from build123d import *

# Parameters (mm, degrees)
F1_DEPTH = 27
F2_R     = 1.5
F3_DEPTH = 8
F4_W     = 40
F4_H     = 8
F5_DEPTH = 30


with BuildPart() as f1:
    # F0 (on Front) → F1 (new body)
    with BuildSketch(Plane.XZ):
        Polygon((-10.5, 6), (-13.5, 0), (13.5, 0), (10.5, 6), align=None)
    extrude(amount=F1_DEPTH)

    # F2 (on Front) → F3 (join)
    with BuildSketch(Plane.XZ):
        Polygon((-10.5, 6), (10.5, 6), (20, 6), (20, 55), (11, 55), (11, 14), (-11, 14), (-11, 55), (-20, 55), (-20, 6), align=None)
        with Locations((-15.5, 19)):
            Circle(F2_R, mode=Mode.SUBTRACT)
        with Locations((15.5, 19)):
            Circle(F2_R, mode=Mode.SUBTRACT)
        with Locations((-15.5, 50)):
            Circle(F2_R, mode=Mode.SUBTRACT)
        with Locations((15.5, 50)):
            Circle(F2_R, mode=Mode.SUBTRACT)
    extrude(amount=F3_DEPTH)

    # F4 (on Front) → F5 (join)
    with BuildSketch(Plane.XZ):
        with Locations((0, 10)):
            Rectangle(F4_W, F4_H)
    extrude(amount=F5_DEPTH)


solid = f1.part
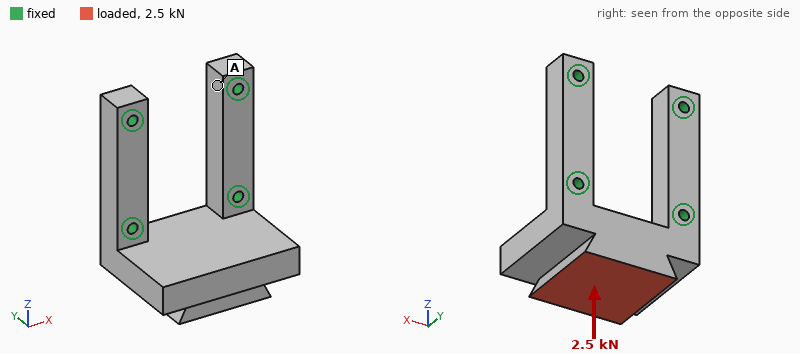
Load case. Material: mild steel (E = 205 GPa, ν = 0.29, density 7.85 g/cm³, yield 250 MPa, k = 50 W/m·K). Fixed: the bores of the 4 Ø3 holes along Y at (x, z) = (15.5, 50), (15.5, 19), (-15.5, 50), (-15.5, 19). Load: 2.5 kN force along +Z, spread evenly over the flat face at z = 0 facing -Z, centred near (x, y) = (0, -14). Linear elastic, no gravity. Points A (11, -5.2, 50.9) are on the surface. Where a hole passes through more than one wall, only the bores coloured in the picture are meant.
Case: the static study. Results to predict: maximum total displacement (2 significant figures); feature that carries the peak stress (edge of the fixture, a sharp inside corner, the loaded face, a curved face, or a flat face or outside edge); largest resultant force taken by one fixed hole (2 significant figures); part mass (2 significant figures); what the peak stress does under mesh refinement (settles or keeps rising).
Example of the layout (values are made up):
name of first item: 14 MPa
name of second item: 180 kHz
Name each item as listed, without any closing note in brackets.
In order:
maximum total displacement: 41 µm
feature that carries the peak stress: edge of the fixture
largest resultant force taken by one fixed hole: 1.3 kN
part mass: 150 g
what the peak stress does under mesh refinement: keeps rising
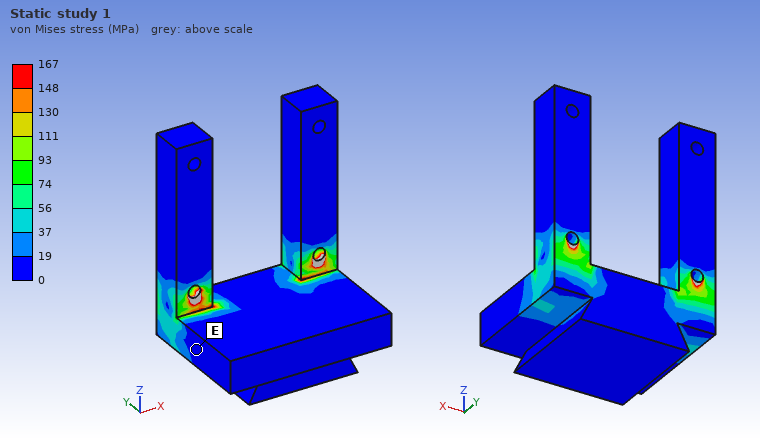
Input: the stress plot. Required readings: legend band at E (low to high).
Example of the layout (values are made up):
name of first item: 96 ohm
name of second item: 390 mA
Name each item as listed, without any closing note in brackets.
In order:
legend band at E: 0 to 19 MPa
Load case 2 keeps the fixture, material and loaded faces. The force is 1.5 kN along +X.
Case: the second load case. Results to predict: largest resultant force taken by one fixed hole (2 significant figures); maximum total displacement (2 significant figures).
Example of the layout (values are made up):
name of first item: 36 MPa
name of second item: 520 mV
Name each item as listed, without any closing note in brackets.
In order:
largest resultant force taken by one fixed hole: 1.2 kN
maximum total displacement: 4.2 µm
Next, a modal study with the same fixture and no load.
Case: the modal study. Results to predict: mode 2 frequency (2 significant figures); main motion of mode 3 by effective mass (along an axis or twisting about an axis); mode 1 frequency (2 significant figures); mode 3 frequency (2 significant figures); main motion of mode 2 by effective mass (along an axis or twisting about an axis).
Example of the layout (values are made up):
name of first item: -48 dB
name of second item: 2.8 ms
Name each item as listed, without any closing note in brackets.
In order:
mode 2 frequency: 10 kHz
main motion of mode 3 by effective mass: along Y
mode 1 frequency: 4000 Hz
mode 3 frequency: 15 kHz
main motion of mode 2 by effective mass: along X
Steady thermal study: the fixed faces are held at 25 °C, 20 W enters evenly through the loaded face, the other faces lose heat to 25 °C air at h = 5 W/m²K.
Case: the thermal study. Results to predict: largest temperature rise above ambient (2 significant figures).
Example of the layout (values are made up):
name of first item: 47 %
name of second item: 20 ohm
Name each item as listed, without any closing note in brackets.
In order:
largest temperature rise above ambient: 38 K
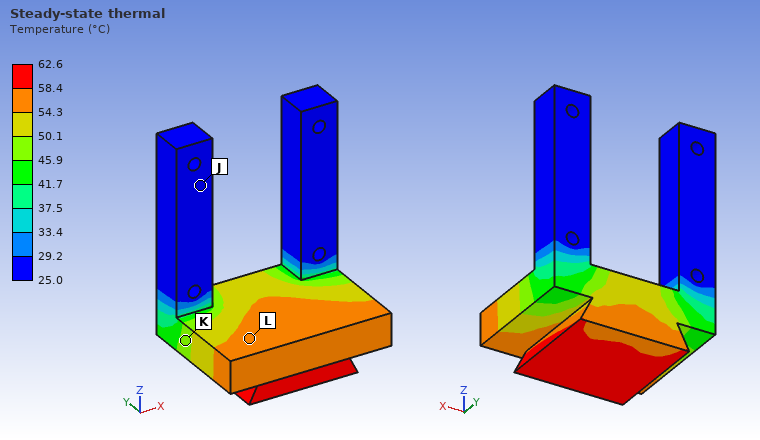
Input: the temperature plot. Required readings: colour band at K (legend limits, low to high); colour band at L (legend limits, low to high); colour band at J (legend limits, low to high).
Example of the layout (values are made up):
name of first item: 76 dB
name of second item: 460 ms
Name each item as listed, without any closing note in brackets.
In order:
colour band at K: 45.9 to 50.1 °C
colour band at L: 54.3 to 58.4 °C
colour band at J: 25.0 to 29.2 °C
